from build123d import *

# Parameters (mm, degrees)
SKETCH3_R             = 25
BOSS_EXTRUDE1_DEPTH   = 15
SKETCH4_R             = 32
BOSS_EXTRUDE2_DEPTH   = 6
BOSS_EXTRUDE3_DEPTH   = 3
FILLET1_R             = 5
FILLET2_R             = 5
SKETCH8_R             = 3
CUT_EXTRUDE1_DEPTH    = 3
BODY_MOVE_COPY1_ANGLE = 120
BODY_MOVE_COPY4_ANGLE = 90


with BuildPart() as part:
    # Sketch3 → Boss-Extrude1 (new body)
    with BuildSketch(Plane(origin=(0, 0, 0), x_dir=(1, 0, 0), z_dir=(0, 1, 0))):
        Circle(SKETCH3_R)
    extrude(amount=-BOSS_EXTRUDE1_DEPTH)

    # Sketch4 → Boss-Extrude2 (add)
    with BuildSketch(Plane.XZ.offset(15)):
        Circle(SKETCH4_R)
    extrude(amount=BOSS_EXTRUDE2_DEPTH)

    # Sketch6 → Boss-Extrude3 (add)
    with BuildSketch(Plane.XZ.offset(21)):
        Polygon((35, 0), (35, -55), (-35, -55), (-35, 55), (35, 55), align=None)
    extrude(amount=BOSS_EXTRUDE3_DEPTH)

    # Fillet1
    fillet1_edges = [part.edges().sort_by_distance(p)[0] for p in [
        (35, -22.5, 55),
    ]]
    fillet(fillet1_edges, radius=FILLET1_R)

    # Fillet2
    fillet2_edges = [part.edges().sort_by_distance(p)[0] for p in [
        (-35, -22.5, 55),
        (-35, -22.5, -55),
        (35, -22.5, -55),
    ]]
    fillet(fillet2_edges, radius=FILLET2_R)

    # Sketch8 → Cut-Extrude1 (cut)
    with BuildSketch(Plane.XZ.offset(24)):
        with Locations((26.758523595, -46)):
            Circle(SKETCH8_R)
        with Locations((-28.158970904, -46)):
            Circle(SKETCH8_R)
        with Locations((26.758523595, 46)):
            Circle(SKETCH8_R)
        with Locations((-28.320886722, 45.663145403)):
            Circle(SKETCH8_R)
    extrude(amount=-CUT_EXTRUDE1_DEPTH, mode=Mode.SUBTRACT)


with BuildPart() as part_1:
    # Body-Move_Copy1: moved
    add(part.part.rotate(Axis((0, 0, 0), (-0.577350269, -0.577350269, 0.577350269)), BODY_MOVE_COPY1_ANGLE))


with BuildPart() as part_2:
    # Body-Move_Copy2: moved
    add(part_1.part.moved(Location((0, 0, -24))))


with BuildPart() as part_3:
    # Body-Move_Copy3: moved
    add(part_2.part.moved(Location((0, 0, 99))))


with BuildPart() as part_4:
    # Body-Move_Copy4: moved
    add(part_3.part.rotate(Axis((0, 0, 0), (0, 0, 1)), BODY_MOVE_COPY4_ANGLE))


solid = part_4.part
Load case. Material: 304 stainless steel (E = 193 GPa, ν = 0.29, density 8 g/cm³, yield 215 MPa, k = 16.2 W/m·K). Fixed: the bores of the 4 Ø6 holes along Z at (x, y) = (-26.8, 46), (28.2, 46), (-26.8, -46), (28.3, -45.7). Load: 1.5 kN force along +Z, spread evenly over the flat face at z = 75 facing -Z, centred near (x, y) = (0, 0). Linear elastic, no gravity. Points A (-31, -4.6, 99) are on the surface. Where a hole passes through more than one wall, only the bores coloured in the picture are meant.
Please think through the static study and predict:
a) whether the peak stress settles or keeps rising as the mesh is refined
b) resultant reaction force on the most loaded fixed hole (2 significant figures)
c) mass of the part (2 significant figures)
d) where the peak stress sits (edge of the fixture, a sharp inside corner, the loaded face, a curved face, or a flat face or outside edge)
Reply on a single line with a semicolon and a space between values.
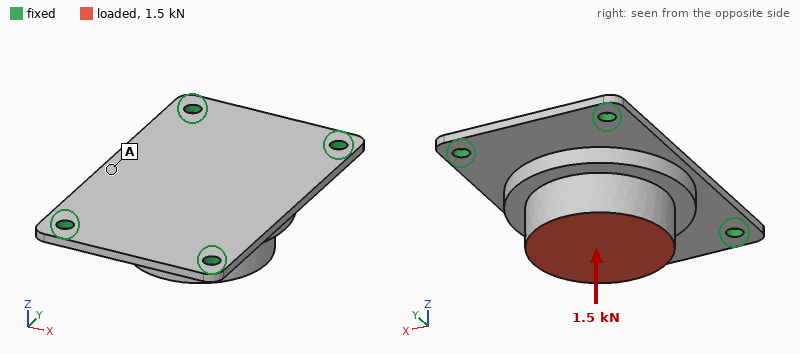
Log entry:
keeps rising; 490 N; 570 g; edge of the fixture
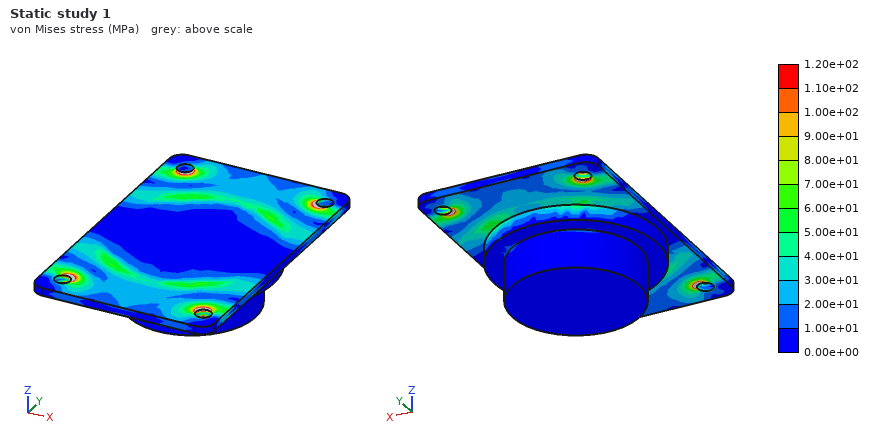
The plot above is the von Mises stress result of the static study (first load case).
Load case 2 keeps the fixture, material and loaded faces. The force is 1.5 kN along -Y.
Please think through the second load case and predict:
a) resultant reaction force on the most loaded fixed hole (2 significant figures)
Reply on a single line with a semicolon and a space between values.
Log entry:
470 N
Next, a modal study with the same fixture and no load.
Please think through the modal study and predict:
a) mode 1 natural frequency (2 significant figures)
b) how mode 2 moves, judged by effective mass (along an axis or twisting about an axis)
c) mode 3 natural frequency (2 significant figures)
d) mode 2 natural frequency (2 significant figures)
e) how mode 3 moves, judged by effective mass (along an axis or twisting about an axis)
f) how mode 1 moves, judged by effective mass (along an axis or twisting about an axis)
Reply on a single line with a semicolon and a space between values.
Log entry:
1600 Hz; along X; 3000 Hz; 1900 Hz; along Y; along Z
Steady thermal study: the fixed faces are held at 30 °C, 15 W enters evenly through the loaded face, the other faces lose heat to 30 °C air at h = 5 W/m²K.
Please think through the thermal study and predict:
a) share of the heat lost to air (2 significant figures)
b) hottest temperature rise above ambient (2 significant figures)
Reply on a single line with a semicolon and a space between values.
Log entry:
24 %; 66 K
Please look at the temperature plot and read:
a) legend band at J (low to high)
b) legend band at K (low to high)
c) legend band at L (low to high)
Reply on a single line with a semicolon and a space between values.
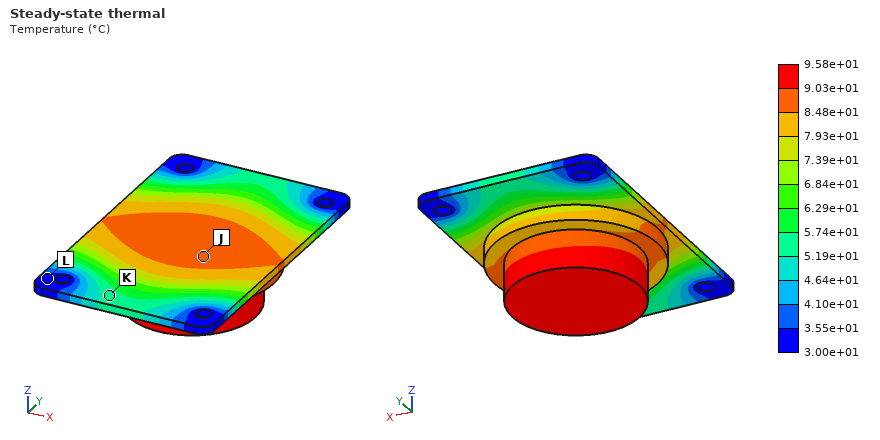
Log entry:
8.48e+01 to 9.03e+01 °C; 5.19e+01 to 5.74e+01 °C; 3.00e+01 to 3.55e+01 °C
